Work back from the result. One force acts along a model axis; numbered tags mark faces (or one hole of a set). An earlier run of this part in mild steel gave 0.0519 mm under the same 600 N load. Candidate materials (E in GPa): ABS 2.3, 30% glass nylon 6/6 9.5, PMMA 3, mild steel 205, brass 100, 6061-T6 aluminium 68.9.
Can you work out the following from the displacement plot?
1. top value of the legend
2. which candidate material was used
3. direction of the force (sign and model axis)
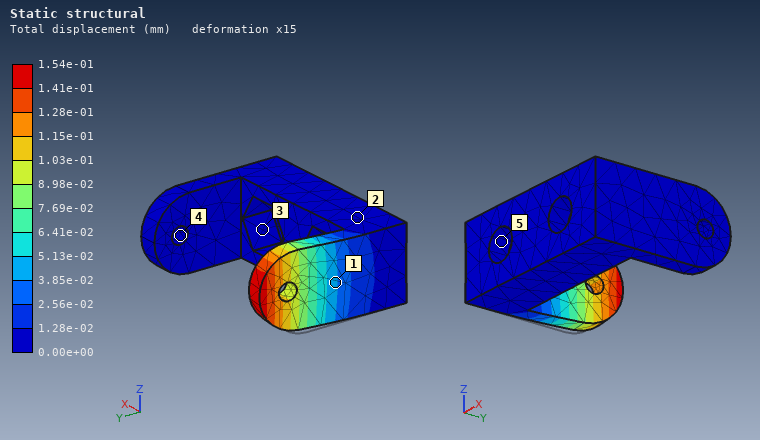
1.54e-01 mm
6061-T6 aluminium
+X
